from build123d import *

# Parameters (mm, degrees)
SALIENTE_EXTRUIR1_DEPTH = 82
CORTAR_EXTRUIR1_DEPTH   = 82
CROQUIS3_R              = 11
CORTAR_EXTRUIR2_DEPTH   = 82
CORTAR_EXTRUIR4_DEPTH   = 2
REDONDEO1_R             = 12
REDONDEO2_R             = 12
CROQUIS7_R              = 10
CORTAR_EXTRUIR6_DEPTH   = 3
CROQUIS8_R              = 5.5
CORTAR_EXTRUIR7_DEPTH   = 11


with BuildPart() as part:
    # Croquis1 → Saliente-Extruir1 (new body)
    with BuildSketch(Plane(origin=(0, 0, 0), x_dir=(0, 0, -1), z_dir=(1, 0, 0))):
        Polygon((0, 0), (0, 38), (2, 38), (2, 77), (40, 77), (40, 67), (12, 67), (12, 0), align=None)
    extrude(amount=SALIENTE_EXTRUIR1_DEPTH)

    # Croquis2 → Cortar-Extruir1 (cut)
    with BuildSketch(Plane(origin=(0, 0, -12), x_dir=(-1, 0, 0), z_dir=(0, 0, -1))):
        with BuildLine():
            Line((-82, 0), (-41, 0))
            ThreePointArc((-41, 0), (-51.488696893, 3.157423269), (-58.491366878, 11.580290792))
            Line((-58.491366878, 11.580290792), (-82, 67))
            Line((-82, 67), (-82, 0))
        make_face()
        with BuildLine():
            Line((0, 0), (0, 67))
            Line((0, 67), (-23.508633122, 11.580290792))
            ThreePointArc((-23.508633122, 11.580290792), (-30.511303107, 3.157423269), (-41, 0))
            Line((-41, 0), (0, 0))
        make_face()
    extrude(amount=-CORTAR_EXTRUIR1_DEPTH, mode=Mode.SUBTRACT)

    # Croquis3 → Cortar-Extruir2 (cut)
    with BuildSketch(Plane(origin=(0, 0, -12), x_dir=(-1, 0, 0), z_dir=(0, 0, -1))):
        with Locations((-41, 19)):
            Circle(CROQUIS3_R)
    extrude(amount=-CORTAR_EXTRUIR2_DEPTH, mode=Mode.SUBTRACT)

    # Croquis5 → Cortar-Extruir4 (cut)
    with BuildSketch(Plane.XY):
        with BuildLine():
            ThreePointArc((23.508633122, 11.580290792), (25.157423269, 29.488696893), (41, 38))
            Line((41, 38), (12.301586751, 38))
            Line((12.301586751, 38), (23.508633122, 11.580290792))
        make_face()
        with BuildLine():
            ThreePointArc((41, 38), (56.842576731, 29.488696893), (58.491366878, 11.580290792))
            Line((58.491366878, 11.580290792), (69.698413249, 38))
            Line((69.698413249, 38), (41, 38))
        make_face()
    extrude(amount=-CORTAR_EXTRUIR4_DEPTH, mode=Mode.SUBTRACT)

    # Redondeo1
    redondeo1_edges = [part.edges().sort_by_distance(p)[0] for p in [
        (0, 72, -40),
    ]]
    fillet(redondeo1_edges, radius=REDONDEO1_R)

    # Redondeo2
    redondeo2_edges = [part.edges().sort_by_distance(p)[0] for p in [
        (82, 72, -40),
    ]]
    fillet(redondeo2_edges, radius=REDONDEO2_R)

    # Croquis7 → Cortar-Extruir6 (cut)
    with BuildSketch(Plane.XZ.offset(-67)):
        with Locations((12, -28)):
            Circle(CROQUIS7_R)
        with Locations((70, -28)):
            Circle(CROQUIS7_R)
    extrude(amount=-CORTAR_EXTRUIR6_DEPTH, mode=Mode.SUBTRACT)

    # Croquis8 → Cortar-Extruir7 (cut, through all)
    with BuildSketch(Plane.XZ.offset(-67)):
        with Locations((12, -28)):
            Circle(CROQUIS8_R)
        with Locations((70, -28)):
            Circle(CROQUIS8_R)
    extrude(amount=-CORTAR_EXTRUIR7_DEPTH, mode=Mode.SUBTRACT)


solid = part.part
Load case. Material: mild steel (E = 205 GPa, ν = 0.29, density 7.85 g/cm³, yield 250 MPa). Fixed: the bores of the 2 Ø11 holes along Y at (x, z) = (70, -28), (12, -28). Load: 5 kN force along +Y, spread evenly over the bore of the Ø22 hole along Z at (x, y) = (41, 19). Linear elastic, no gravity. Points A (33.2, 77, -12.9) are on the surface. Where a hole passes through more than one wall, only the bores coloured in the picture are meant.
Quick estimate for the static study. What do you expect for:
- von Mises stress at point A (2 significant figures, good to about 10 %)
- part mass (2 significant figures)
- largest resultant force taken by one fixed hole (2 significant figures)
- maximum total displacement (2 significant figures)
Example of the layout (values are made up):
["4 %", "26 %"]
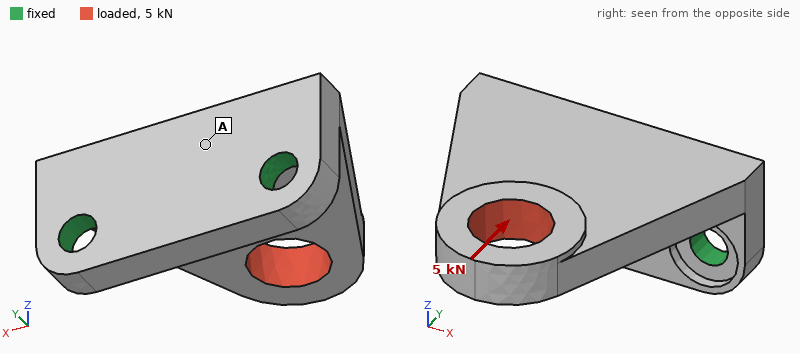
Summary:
["25 MPa", "470 g", "2.5 kN", "0.11 mm"]
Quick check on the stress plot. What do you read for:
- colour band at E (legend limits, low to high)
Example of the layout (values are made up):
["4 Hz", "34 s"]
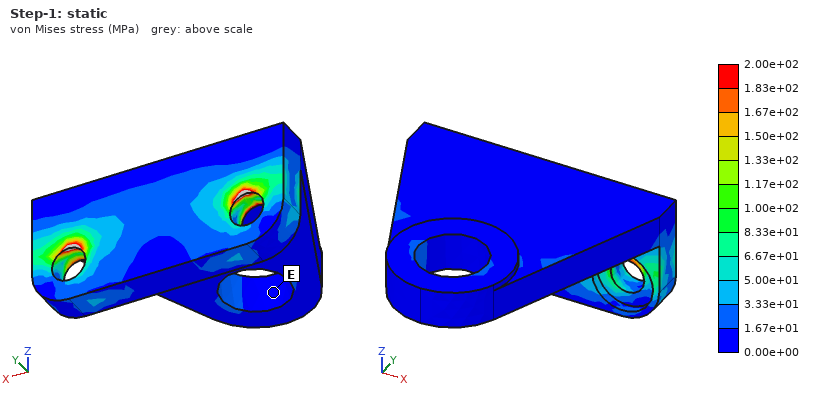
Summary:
["0.00e+00 to 1.67e+01 MPa"]
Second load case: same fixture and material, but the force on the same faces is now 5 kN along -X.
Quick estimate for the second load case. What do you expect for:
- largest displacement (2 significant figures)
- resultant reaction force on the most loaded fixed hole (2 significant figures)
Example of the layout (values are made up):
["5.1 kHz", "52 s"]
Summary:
["62 µm", "5.4 kN"]
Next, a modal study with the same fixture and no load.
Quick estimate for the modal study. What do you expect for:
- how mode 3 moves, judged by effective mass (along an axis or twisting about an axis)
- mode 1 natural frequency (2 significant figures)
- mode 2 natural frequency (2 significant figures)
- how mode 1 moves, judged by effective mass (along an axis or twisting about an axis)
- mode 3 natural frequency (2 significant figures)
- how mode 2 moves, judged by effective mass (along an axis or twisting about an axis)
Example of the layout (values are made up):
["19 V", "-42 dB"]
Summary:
["along Y", "1500 Hz", "4300 Hz", "along Z", "5500 Hz", "along X"]
